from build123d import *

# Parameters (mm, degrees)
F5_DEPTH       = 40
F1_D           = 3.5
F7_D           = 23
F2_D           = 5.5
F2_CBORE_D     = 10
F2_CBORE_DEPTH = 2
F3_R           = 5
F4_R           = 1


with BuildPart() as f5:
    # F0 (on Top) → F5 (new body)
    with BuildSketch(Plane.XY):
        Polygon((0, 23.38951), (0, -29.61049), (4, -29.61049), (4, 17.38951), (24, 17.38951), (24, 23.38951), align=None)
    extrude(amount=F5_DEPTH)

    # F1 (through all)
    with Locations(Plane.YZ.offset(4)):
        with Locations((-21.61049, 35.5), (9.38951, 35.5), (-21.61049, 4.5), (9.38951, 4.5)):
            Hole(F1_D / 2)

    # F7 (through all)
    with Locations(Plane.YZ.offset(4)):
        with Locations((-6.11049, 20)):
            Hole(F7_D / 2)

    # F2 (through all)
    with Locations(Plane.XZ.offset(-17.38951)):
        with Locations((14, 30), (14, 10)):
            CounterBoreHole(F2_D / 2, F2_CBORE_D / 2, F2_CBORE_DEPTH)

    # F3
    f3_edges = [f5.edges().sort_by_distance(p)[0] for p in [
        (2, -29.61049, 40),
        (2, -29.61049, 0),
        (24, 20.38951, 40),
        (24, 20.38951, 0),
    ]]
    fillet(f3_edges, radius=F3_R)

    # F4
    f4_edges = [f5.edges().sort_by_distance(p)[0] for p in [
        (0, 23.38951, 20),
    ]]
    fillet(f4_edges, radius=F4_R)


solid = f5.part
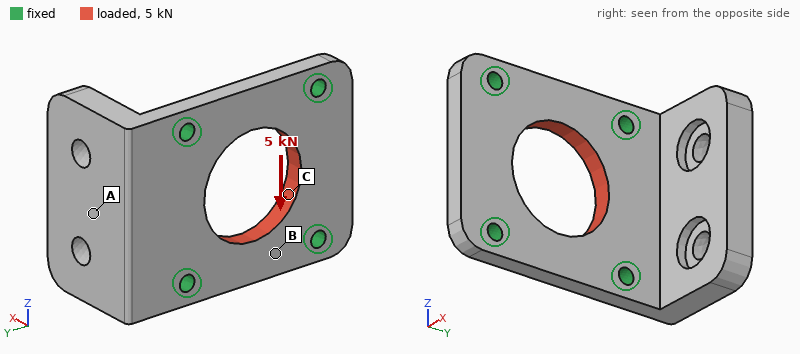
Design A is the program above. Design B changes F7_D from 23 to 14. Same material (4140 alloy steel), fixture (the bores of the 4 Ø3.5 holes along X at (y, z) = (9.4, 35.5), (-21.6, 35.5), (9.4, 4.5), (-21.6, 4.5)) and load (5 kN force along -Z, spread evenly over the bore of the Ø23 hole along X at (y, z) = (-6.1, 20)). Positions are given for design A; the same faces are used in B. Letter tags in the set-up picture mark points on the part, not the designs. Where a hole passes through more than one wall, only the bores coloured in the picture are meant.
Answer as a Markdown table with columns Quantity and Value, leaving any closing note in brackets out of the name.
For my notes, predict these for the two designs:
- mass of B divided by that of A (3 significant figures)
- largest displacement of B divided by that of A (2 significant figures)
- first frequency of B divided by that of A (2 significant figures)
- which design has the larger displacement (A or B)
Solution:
| Quantity | Value |
|---|---|
| mass of B divided by that of A | 1.10 |
| largest displacement of B divided by that of A | 0.87 |
| first frequency of B divided by that of A | 1.0 |
| which design has the larger displacement | A |
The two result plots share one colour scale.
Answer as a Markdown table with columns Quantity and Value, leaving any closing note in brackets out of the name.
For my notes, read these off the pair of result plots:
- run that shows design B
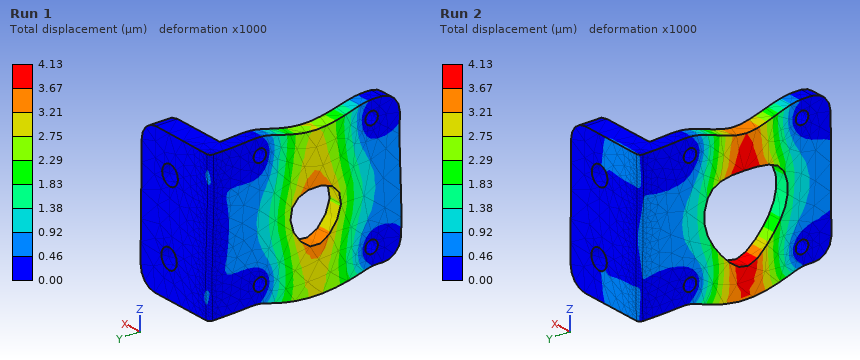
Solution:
| Quantity | Value |
|---|---|
| run that shows design B | Run 1 |
